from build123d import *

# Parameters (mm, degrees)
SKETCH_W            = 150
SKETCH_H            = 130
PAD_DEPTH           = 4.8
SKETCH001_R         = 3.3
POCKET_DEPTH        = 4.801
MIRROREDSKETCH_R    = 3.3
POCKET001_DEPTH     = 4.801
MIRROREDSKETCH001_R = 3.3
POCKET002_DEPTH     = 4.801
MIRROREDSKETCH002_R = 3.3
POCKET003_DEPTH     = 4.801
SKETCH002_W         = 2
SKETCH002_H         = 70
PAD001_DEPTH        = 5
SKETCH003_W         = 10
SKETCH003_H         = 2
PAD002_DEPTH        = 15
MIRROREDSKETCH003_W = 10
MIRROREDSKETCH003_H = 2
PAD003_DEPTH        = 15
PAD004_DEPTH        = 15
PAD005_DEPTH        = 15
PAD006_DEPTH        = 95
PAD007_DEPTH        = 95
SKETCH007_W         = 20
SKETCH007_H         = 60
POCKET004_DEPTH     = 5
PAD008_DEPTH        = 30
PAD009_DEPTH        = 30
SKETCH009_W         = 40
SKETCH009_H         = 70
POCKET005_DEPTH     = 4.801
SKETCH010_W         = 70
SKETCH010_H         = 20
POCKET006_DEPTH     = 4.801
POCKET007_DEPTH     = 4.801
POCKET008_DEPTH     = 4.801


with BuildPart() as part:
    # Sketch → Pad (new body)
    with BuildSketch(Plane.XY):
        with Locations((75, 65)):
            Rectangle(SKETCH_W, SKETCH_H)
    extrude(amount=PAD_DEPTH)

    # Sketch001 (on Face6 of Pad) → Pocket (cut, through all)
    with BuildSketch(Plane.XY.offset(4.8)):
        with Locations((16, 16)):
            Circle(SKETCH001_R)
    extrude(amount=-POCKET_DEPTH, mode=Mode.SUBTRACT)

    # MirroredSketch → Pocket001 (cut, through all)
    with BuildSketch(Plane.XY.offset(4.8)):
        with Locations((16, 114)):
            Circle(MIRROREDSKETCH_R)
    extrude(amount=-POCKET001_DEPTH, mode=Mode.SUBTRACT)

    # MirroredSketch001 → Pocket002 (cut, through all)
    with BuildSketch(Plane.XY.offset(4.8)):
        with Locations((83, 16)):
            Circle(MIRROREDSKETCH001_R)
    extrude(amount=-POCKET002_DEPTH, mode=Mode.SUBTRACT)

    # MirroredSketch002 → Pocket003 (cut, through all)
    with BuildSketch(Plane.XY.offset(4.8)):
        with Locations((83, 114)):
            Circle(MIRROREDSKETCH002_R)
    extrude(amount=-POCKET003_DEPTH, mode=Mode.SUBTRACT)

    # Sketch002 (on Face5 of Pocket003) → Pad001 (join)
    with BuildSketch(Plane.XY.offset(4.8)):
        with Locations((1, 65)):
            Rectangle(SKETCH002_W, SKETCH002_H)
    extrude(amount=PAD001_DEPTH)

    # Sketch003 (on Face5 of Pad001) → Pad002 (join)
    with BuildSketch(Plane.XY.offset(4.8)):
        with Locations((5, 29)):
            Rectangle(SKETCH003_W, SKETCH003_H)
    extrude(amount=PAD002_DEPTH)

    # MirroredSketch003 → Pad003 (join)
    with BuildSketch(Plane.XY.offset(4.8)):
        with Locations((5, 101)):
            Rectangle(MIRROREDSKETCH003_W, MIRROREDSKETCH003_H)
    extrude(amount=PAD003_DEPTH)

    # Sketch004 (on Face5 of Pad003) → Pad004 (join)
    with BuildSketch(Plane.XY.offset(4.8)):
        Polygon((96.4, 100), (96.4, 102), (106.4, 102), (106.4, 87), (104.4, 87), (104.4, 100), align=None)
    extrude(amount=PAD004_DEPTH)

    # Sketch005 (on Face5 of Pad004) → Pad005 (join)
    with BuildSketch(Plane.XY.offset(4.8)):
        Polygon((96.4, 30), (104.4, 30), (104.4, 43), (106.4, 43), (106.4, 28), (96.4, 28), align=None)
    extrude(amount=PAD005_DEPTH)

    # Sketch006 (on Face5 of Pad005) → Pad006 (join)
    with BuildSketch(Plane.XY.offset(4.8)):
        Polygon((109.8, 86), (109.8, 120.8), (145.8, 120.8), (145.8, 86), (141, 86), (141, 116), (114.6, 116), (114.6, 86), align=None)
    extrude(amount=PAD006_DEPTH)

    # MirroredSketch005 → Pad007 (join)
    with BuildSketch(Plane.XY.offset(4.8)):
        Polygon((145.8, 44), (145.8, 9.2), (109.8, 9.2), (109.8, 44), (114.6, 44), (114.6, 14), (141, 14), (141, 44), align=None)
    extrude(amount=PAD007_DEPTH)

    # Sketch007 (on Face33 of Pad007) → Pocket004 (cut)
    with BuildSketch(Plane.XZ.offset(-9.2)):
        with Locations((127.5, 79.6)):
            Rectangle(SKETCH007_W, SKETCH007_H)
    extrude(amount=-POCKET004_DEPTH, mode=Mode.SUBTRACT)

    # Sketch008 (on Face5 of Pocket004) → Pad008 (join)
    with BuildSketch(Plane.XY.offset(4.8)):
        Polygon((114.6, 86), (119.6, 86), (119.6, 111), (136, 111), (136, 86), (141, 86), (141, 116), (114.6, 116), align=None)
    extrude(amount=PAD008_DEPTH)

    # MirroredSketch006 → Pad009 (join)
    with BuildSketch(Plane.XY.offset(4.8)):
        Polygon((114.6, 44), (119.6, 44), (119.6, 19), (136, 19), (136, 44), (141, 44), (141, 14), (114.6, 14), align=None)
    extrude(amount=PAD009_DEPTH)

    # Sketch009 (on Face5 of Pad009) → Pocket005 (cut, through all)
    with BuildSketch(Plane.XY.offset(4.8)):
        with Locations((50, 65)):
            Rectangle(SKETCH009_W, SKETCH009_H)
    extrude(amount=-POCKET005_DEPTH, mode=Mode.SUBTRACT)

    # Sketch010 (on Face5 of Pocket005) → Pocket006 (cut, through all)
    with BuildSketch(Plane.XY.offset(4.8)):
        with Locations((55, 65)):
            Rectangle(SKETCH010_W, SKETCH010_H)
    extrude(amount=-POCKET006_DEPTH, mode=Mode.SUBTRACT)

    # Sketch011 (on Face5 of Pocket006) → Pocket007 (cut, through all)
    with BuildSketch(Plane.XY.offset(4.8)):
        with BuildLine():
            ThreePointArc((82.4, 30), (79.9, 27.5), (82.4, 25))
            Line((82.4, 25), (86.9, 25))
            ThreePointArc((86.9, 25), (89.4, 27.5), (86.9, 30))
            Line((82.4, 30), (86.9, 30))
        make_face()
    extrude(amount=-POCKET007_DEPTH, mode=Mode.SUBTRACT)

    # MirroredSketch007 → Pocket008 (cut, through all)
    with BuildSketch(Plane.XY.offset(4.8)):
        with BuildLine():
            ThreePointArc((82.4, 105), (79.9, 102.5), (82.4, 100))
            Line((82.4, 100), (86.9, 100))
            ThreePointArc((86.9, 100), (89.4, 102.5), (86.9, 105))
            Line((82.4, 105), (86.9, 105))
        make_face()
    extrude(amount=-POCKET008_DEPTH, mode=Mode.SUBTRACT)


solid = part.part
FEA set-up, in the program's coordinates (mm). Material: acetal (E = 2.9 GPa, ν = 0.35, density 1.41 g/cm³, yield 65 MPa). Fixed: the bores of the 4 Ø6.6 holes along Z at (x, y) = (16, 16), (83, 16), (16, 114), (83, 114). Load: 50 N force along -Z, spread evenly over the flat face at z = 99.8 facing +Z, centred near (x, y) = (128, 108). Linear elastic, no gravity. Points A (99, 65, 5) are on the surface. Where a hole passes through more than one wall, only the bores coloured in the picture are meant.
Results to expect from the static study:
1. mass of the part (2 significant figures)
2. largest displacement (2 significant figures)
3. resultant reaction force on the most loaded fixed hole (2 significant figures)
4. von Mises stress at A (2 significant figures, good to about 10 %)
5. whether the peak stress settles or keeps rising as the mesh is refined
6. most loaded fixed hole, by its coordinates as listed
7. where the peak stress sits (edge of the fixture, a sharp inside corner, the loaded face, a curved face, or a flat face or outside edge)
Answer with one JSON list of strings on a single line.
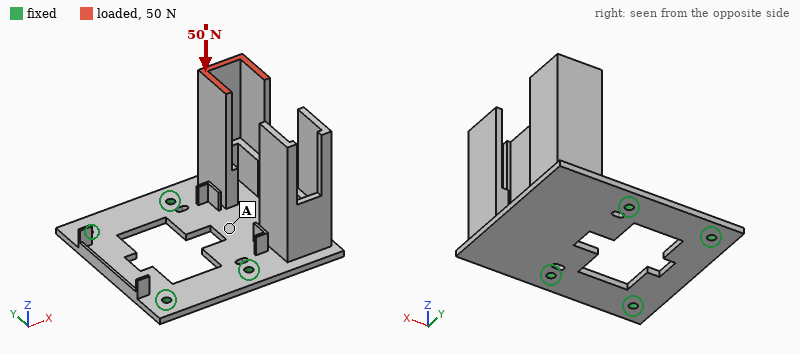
["260 g", "2.3 mm", "48 N", "1.3 MPa", "keeps rising", "(83, 114)", "edge of the fixture"]
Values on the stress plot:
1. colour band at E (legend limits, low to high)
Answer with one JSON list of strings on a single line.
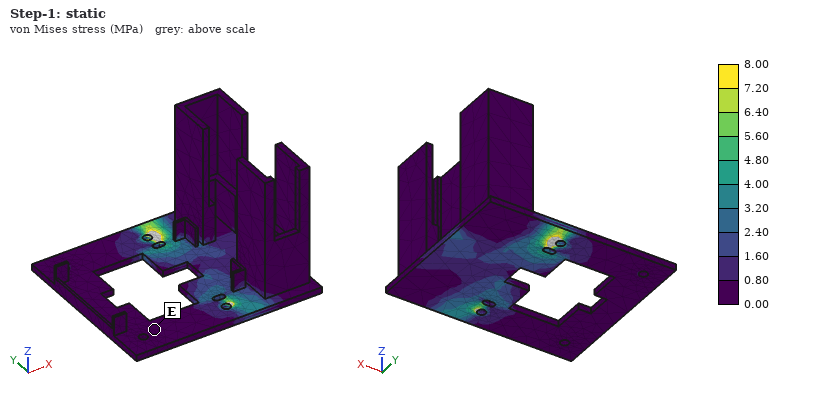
["0.00 to 0.80 MPa"]
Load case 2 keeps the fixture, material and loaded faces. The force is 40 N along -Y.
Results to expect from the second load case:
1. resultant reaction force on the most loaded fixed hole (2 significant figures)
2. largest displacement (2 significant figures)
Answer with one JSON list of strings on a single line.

["45 N", "2.1 mm"]
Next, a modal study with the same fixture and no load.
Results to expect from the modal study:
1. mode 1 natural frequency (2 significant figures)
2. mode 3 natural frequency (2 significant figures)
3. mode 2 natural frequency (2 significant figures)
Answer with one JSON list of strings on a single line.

["61 Hz", "130 Hz", "120 Hz"]
